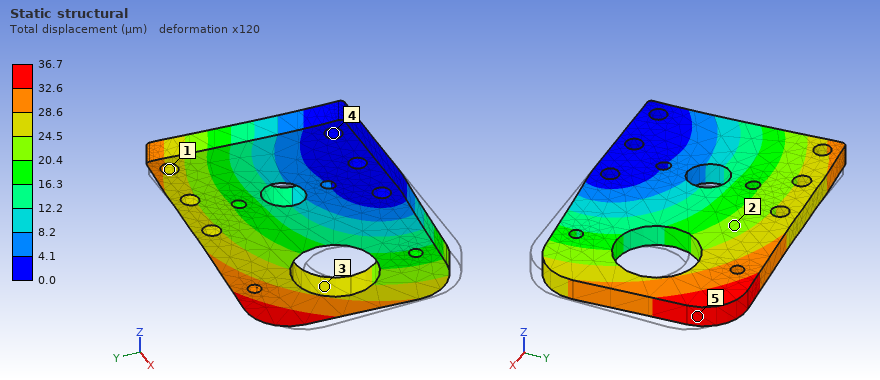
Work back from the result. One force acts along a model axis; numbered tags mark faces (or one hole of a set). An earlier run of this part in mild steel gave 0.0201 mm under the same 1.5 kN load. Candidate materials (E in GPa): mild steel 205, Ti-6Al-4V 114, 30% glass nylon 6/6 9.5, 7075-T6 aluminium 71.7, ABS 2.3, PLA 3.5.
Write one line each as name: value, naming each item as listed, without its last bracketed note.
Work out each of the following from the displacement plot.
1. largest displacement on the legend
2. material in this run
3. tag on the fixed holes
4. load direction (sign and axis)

largest displacement on the legend: 36.7 µm
material in this run: Ti-6Al-4V
tag on the fixed holes: 4
load direction: -X
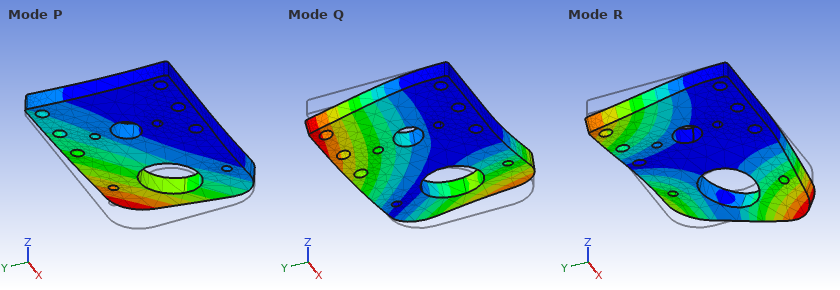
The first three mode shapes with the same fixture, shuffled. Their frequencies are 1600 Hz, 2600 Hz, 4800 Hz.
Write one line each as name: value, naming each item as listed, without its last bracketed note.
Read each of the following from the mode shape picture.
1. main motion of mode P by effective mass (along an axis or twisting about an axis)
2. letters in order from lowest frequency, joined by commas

main motion of mode P by effective mass: along Z
letters in order from lowest frequency, joined by commas: P, Q, R
